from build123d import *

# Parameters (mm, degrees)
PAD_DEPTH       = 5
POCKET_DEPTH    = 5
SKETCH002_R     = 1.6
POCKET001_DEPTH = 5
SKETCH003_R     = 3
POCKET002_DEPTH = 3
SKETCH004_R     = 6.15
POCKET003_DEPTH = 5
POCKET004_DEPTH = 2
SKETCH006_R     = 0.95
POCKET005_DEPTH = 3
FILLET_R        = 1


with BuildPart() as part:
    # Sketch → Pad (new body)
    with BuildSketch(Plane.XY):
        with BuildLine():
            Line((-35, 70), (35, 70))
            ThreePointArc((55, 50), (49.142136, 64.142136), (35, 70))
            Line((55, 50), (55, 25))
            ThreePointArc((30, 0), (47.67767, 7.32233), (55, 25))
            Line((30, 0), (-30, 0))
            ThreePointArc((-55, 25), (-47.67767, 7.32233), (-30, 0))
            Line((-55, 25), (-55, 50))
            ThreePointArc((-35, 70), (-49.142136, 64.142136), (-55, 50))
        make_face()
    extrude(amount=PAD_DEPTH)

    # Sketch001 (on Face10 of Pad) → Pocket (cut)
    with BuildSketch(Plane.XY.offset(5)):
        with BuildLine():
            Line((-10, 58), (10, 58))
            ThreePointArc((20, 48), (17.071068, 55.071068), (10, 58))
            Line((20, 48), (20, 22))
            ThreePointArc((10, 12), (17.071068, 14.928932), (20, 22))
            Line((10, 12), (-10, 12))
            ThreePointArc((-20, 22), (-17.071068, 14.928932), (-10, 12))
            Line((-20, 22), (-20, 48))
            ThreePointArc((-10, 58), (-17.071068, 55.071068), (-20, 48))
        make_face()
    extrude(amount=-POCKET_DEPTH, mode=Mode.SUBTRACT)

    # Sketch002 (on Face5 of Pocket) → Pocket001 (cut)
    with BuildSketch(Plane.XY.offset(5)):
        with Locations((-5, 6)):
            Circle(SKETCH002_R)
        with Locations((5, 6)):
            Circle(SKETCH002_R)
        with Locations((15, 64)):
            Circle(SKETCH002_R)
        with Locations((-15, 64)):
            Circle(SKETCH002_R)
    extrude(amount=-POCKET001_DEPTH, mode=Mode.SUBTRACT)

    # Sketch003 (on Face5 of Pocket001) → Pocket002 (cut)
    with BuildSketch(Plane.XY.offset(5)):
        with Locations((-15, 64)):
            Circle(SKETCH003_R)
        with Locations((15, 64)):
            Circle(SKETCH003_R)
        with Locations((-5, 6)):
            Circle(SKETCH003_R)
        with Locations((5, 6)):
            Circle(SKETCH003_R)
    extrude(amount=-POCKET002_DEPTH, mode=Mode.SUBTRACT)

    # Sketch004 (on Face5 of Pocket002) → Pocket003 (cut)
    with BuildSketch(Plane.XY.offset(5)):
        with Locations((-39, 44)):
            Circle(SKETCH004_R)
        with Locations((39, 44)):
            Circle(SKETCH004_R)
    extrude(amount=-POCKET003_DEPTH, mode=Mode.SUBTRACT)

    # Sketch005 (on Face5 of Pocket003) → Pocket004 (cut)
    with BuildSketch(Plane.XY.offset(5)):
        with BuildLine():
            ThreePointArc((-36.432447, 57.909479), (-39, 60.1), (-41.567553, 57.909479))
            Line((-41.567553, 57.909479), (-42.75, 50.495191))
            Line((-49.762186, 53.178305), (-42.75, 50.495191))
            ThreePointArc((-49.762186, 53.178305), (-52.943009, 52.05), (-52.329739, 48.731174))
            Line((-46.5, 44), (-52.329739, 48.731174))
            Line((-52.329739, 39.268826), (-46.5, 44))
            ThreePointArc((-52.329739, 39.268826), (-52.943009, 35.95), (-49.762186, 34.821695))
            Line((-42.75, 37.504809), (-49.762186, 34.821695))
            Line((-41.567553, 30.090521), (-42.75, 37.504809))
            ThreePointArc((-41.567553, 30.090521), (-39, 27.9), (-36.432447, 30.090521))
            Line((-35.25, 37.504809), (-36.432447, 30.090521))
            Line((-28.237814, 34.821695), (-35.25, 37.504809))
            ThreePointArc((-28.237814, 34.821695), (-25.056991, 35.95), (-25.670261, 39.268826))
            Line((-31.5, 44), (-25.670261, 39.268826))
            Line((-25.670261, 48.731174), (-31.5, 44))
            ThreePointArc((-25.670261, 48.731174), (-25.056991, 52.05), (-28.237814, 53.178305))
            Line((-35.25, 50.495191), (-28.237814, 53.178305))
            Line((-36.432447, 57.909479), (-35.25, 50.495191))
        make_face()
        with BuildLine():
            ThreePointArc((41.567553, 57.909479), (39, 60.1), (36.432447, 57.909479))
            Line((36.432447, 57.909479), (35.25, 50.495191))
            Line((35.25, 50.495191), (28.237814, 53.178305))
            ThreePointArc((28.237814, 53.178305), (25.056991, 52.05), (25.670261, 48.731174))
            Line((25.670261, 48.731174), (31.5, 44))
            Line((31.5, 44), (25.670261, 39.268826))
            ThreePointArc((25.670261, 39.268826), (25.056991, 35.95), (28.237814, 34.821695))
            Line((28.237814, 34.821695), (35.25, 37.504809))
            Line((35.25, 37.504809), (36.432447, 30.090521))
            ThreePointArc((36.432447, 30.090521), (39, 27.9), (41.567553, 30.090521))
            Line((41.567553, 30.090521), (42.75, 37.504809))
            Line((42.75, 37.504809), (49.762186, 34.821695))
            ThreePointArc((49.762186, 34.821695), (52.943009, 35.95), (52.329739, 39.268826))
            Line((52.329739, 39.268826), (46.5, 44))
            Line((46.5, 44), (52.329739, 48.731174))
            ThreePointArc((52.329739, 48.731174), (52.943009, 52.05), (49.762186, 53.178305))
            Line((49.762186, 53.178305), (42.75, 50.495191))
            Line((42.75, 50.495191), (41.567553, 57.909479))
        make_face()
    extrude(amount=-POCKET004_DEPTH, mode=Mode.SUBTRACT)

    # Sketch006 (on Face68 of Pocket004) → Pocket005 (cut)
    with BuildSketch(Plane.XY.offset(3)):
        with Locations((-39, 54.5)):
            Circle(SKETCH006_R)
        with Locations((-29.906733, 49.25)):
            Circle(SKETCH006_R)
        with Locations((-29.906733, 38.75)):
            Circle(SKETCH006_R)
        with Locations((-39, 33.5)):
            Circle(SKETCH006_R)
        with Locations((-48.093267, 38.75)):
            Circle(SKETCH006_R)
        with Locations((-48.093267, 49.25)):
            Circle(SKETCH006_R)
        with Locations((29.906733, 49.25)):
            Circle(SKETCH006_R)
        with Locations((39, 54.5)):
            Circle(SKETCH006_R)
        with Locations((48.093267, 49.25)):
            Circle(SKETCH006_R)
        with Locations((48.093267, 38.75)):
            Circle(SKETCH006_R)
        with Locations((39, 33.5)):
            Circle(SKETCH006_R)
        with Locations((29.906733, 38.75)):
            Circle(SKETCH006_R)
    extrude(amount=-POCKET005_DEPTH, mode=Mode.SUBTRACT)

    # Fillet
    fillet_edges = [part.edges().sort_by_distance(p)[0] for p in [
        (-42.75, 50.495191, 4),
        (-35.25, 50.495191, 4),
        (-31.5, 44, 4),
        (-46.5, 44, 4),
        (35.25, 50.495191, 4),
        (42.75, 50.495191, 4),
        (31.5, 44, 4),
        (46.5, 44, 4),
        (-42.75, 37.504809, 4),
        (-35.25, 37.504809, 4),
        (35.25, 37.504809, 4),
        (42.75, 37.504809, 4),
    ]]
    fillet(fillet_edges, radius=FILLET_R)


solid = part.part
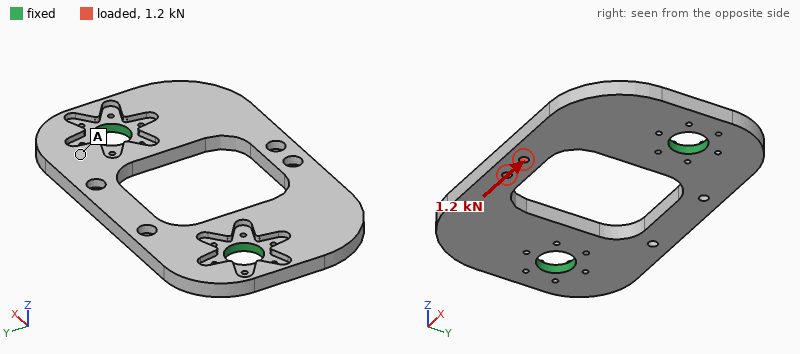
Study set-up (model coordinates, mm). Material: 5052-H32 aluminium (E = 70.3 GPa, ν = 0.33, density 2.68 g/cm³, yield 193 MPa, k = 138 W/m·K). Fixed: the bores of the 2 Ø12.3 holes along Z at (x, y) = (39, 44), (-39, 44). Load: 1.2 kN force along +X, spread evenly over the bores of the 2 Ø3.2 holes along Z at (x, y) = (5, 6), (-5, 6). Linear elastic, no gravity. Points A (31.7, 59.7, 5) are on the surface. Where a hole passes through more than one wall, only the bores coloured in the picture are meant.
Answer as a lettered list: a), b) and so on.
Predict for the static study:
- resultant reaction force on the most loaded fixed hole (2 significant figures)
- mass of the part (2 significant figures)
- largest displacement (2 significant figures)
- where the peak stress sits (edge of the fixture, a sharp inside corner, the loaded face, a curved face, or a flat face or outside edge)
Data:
a) 670 N
b) 65 g
c) 31 µm
d) the loaded face
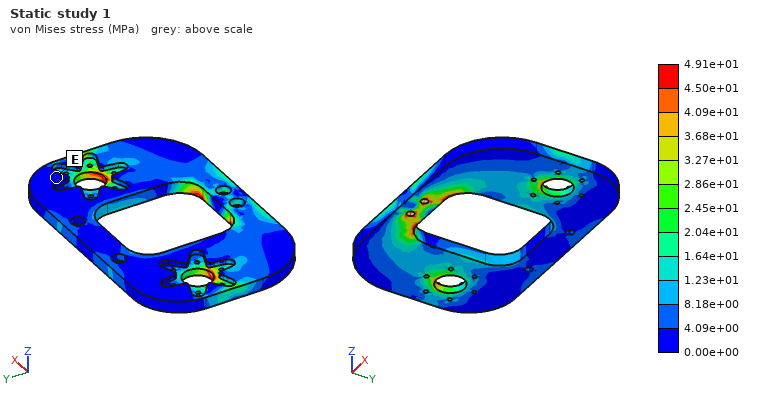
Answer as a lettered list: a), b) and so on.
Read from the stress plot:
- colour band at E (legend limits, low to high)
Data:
a) 0.00e+00 to 4.09e+00 MPa
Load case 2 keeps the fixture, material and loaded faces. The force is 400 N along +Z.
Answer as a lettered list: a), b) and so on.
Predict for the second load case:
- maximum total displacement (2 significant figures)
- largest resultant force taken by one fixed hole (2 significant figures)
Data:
a) 0.41 mm
b) 210 N
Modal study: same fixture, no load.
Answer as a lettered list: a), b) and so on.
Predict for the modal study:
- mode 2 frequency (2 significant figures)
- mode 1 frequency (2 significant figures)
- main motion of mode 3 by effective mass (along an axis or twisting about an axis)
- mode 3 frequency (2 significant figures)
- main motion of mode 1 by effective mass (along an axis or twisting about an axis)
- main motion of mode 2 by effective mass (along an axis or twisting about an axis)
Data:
a) 2700 Hz
b) 1600 Hz
c) along Z
d) 3300 Hz
e) along Z
f) twisting about Y
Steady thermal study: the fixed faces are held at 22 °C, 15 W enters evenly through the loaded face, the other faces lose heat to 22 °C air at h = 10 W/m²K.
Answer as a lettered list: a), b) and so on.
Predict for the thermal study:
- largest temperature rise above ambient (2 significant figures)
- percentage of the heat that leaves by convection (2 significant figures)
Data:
a) 35 K
b) 5.8 %
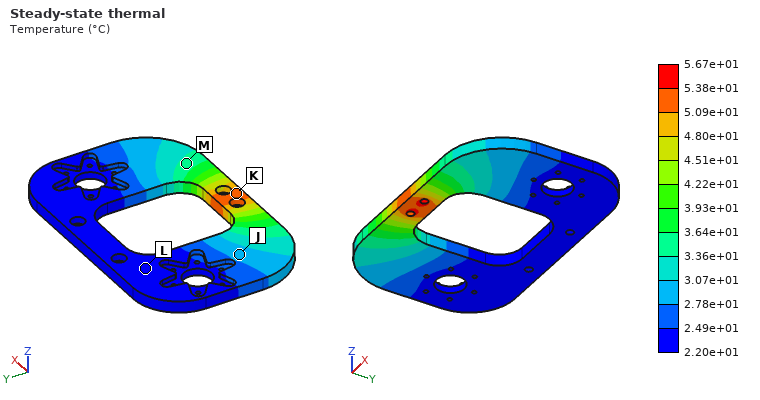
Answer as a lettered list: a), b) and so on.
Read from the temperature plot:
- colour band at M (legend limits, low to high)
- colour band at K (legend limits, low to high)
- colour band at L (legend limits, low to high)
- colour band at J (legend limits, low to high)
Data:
a) 3.36e+01 to 3.64e+01 °C
b) 5.09e+01 to 5.38e+01 °C
c) 2.20e+01 to 2.49e+01 °C
d) 2.78e+01 to 3.07e+01 °C
